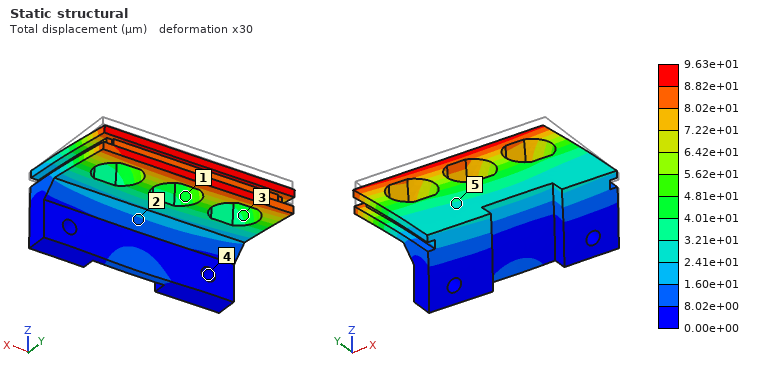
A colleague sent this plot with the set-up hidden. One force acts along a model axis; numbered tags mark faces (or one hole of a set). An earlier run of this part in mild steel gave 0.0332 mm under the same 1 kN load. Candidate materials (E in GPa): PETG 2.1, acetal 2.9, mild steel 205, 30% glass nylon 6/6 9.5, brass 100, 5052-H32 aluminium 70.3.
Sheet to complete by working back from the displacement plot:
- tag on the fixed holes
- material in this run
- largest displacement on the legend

4
5052-H32 aluminium
9.63e+01 µm
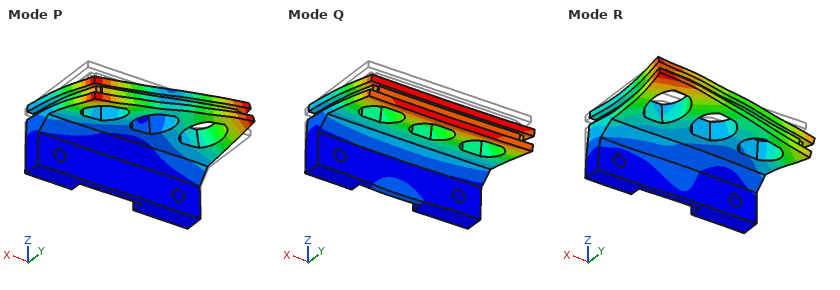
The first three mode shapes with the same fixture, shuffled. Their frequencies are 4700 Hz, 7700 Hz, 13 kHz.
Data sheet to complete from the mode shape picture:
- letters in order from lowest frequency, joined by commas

Q, P, R
